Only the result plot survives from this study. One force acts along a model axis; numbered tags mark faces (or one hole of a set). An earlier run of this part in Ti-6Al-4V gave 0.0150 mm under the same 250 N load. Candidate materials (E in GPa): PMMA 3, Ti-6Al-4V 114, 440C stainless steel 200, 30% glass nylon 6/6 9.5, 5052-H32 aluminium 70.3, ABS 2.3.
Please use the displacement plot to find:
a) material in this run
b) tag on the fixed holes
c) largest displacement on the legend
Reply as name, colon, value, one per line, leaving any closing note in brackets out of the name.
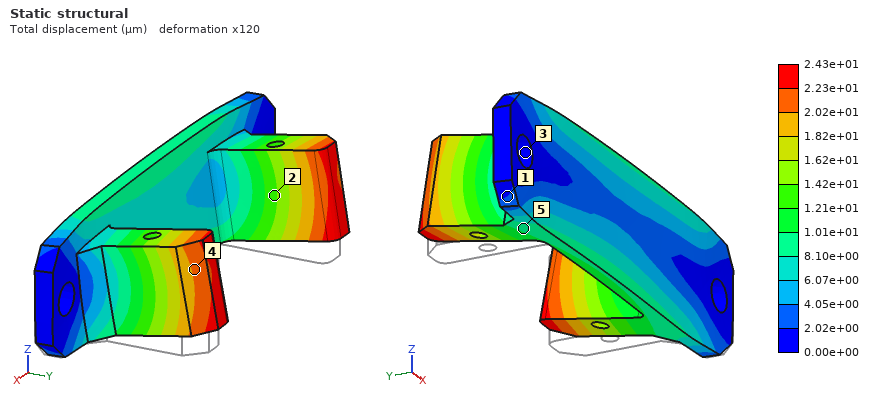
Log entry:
material in this run: 5052-H32 aluminium
tag on the fixed holes: 3
largest displacement on the legend: 2.43e+01 µm
